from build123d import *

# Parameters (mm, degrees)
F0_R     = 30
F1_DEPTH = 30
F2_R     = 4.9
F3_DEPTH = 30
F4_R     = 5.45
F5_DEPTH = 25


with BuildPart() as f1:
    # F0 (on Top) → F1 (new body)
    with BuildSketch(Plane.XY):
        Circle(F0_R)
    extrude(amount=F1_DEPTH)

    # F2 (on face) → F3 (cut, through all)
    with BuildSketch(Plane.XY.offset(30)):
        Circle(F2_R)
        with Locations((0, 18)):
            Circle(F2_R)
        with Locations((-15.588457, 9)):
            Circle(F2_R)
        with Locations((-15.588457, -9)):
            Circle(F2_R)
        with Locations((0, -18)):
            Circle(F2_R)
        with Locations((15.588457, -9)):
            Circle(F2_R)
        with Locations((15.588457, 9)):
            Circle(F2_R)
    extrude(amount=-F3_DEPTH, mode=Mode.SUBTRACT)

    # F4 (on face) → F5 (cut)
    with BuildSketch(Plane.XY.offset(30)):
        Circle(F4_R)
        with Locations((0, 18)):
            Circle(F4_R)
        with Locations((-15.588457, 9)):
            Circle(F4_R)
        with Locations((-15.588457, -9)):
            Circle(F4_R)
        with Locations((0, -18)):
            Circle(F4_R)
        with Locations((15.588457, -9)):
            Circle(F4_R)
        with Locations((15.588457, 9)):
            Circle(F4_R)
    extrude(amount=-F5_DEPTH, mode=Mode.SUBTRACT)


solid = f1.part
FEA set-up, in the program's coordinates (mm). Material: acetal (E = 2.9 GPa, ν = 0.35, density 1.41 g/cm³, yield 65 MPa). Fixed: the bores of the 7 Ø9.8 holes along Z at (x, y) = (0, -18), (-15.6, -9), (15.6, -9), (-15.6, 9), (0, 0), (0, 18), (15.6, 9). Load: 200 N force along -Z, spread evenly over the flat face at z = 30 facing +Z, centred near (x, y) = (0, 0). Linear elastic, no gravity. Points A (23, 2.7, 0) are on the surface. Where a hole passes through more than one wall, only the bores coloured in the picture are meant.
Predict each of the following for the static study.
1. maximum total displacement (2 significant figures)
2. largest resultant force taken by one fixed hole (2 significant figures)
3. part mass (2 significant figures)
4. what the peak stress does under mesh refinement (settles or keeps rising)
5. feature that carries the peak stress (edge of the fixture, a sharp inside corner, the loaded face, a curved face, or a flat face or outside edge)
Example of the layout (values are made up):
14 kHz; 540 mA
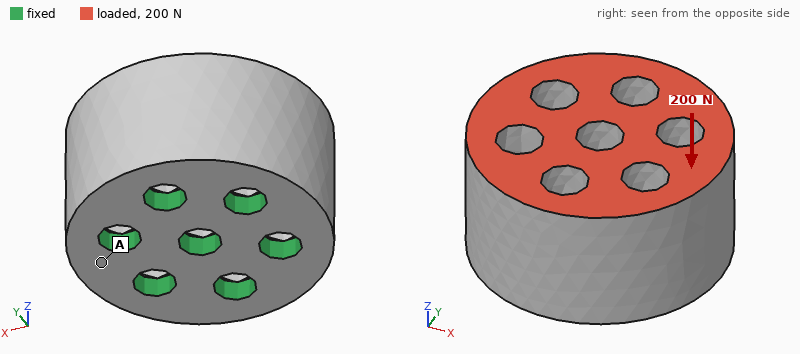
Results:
1.6 µm; 30 N; 93 g; keeps rising; edge of the fixture
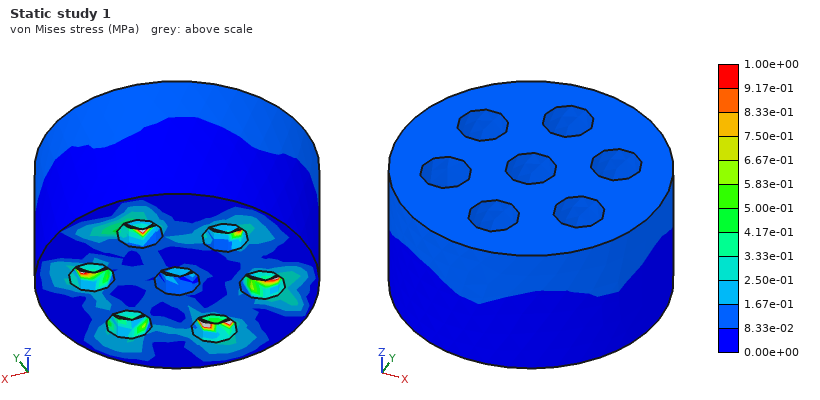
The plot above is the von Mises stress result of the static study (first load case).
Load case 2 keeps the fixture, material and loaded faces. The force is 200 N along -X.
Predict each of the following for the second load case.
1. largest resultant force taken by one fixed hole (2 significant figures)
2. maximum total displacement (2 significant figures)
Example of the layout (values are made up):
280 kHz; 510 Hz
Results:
79 N; 10 µm
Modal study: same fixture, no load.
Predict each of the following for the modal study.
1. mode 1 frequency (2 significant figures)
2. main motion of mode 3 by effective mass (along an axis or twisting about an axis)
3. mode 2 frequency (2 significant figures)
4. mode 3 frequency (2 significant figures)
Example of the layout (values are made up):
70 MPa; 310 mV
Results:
4200 Hz; twisting about Z; 4200 Hz; 6400 Hz
